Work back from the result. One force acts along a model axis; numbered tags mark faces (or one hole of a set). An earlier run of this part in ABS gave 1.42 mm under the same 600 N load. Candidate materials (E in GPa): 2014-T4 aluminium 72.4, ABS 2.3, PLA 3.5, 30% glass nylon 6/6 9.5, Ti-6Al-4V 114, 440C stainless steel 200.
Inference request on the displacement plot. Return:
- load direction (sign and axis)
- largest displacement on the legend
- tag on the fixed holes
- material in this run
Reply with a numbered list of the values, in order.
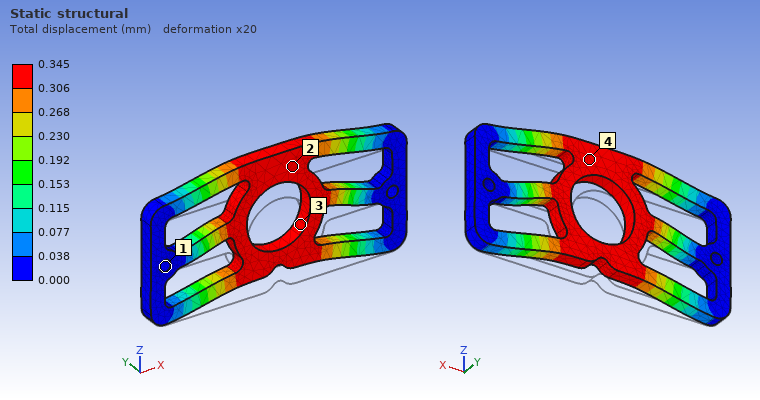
1. +Z
2. 0.345 mm
3. 1
4. 30% glass nylon 6/6
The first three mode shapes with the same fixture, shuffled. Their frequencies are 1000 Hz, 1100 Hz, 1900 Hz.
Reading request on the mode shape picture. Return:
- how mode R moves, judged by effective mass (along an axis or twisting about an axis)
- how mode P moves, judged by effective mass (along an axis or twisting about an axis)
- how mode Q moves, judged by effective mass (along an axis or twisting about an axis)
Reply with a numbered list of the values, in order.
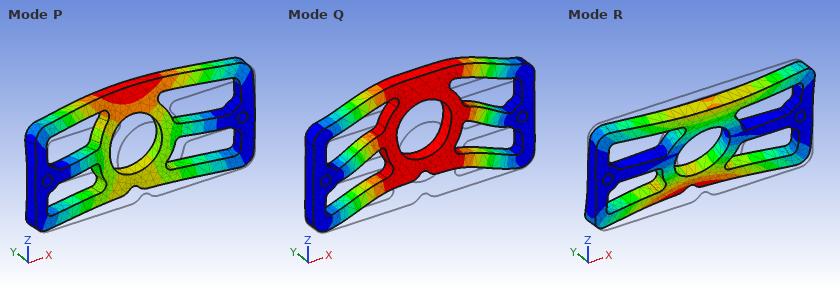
1. twisting about X
2. along Y
3. along Z
